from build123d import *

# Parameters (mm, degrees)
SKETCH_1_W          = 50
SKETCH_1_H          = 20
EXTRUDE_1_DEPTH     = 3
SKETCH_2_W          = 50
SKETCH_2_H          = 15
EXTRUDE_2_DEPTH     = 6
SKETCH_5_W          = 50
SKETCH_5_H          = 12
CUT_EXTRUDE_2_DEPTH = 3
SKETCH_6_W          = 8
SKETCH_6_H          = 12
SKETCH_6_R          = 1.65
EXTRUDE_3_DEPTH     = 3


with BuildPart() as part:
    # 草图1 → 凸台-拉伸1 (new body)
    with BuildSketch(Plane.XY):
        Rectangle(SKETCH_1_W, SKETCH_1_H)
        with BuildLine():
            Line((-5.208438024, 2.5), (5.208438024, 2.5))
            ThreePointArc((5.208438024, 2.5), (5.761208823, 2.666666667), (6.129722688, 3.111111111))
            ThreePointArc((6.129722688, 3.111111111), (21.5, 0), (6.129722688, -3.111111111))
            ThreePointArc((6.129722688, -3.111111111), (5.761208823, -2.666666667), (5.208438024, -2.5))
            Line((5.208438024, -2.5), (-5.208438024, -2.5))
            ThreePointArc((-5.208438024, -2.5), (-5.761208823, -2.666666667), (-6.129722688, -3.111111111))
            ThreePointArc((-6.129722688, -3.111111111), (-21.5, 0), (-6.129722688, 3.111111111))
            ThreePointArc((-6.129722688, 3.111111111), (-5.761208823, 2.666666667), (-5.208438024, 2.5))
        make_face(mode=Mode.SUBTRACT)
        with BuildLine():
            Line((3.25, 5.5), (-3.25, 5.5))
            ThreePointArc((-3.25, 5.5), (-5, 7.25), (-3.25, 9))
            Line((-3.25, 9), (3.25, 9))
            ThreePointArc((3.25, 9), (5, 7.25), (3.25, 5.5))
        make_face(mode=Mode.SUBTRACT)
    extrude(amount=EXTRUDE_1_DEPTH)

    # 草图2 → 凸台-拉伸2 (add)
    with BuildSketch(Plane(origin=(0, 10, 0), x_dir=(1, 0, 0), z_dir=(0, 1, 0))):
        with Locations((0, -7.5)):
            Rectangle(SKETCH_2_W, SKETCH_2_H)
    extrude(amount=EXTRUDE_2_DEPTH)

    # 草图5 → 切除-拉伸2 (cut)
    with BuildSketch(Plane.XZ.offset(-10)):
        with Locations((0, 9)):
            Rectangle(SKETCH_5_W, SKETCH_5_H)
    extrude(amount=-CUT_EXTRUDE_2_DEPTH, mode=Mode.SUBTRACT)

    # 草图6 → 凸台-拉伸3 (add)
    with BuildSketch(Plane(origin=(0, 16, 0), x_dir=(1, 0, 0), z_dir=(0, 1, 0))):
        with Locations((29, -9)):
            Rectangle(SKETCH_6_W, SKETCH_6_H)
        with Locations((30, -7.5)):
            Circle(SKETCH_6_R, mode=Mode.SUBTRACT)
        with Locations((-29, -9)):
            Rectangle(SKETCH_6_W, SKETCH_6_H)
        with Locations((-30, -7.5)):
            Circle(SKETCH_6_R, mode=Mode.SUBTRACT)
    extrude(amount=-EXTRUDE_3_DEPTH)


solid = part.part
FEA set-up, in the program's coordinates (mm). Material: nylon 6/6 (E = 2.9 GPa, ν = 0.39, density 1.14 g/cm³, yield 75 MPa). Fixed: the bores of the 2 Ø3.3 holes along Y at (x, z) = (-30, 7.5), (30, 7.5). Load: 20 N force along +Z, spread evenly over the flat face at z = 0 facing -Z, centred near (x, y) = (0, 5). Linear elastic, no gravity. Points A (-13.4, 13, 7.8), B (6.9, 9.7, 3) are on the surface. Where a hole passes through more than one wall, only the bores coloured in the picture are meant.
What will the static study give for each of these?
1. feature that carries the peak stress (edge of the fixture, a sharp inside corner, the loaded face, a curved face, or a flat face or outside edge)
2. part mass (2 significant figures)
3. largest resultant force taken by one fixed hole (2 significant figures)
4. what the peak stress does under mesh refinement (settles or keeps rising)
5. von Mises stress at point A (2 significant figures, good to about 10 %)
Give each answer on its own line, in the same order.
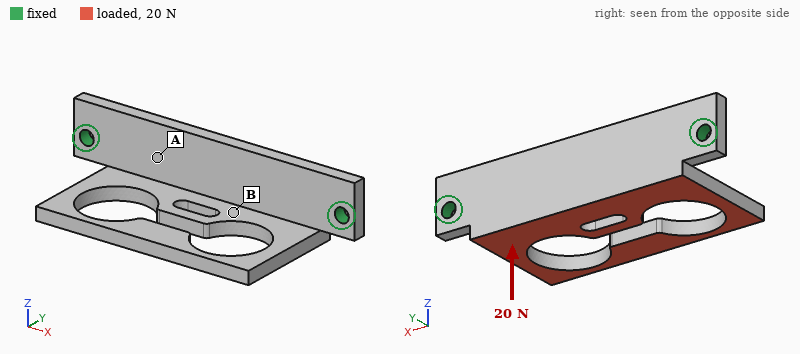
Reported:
edge of the fixture
5.4 g
10 N
keeps rising
1.9 MPa
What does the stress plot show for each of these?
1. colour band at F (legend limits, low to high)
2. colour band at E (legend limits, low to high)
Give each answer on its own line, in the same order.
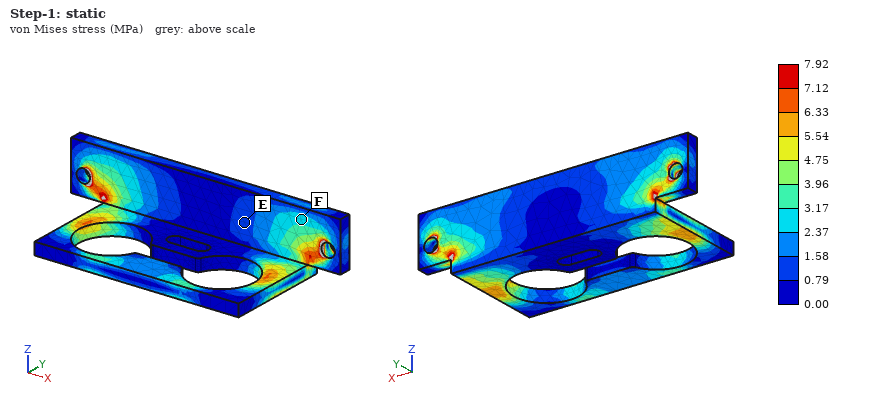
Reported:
2.37 to 3.17 MPa
0.79 to 1.58 MPa
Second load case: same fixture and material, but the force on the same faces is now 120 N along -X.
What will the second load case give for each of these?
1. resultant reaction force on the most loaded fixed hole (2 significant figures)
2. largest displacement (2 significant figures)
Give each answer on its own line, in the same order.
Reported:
66 N
0.61 mm
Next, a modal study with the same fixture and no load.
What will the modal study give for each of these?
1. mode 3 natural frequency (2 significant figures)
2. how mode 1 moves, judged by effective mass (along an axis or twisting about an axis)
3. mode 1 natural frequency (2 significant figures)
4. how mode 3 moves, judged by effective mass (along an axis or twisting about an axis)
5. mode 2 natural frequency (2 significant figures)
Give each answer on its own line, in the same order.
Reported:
1500 Hz
along Z
600 Hz
along X
1300 Hz
